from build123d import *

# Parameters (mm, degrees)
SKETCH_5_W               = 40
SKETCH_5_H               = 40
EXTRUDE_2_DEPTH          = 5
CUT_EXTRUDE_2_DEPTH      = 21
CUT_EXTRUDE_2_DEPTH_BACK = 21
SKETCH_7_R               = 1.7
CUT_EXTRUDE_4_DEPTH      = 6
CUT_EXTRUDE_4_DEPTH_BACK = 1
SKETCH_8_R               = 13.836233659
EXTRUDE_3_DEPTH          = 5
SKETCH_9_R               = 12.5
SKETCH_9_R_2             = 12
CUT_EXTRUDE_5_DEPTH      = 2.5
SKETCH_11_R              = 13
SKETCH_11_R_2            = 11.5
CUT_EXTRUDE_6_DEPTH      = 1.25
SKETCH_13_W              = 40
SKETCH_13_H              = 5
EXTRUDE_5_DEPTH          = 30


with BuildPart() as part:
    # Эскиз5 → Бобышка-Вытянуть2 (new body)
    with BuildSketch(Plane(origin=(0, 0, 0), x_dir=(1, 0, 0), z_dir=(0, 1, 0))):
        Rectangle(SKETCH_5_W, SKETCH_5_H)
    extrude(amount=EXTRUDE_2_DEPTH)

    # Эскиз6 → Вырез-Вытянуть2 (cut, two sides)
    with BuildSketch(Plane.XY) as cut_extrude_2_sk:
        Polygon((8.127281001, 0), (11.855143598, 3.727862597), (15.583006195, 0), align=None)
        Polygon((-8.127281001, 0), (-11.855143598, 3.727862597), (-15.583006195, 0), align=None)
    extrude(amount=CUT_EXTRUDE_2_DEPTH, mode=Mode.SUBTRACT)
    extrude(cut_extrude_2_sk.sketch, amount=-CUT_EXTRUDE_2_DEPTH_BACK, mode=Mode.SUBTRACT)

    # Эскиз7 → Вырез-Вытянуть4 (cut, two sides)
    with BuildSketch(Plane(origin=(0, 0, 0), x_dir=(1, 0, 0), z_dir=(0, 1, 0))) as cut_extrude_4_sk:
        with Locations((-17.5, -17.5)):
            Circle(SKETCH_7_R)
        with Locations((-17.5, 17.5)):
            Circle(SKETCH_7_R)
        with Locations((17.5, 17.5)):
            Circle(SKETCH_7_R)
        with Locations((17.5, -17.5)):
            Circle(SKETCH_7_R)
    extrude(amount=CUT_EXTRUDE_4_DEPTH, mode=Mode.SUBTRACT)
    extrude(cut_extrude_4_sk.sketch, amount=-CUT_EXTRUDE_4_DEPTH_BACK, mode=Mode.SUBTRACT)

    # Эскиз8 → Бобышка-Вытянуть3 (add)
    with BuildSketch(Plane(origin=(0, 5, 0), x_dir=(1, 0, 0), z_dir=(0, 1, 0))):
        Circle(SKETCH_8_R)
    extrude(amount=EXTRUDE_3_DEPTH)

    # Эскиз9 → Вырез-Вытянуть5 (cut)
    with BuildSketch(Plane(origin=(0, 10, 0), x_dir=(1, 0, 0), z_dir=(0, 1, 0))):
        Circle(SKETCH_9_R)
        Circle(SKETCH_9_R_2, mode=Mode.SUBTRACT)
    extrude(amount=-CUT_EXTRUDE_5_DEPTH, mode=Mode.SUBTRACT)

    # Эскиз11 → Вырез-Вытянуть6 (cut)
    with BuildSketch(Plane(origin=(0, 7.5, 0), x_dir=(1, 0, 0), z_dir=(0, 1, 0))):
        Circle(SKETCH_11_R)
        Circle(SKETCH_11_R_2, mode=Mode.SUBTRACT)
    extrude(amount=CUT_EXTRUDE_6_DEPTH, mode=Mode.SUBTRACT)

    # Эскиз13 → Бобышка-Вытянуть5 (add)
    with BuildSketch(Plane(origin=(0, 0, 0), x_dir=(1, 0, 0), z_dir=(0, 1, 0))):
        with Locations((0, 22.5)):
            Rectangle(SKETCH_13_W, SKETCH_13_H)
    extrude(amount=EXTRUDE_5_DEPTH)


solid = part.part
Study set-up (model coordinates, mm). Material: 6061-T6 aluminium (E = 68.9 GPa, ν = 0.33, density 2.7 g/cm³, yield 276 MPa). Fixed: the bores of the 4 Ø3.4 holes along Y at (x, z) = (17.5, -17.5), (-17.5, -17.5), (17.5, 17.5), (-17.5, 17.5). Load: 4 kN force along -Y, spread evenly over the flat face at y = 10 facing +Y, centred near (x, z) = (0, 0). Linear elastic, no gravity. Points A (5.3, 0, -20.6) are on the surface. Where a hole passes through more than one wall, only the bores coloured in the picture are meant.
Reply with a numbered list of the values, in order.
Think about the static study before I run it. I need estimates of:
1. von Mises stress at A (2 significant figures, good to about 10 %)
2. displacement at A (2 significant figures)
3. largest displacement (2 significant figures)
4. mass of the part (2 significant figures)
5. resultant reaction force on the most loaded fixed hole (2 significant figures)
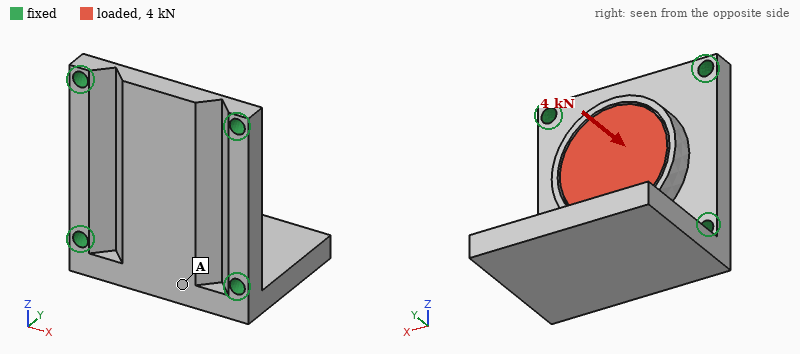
1. 21 MPa
2. 10 µm
3. 42 µm
4. 42 g
5. 1.1 kN
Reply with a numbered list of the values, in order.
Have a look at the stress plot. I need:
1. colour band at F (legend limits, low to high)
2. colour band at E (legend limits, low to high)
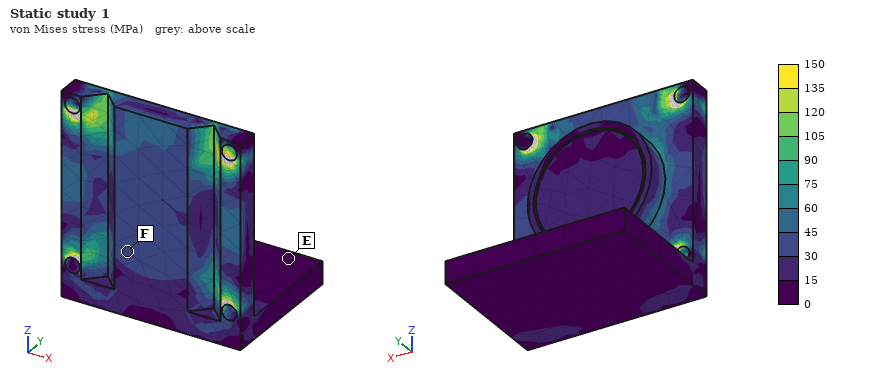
1. 30 to 45 MPa
2. 0 to 15 MPa
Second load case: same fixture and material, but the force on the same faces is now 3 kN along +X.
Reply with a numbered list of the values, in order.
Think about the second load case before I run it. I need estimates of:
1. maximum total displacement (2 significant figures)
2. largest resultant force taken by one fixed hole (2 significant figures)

1. 19 µm
2. 950 N
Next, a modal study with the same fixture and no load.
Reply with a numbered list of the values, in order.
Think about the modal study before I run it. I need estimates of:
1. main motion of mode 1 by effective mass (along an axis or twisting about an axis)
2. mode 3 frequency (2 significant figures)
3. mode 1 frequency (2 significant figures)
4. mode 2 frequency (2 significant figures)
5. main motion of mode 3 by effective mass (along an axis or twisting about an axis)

1. along Z
2. 12 kHz
3. 4000 Hz
4. 8600 Hz
5. along Y
